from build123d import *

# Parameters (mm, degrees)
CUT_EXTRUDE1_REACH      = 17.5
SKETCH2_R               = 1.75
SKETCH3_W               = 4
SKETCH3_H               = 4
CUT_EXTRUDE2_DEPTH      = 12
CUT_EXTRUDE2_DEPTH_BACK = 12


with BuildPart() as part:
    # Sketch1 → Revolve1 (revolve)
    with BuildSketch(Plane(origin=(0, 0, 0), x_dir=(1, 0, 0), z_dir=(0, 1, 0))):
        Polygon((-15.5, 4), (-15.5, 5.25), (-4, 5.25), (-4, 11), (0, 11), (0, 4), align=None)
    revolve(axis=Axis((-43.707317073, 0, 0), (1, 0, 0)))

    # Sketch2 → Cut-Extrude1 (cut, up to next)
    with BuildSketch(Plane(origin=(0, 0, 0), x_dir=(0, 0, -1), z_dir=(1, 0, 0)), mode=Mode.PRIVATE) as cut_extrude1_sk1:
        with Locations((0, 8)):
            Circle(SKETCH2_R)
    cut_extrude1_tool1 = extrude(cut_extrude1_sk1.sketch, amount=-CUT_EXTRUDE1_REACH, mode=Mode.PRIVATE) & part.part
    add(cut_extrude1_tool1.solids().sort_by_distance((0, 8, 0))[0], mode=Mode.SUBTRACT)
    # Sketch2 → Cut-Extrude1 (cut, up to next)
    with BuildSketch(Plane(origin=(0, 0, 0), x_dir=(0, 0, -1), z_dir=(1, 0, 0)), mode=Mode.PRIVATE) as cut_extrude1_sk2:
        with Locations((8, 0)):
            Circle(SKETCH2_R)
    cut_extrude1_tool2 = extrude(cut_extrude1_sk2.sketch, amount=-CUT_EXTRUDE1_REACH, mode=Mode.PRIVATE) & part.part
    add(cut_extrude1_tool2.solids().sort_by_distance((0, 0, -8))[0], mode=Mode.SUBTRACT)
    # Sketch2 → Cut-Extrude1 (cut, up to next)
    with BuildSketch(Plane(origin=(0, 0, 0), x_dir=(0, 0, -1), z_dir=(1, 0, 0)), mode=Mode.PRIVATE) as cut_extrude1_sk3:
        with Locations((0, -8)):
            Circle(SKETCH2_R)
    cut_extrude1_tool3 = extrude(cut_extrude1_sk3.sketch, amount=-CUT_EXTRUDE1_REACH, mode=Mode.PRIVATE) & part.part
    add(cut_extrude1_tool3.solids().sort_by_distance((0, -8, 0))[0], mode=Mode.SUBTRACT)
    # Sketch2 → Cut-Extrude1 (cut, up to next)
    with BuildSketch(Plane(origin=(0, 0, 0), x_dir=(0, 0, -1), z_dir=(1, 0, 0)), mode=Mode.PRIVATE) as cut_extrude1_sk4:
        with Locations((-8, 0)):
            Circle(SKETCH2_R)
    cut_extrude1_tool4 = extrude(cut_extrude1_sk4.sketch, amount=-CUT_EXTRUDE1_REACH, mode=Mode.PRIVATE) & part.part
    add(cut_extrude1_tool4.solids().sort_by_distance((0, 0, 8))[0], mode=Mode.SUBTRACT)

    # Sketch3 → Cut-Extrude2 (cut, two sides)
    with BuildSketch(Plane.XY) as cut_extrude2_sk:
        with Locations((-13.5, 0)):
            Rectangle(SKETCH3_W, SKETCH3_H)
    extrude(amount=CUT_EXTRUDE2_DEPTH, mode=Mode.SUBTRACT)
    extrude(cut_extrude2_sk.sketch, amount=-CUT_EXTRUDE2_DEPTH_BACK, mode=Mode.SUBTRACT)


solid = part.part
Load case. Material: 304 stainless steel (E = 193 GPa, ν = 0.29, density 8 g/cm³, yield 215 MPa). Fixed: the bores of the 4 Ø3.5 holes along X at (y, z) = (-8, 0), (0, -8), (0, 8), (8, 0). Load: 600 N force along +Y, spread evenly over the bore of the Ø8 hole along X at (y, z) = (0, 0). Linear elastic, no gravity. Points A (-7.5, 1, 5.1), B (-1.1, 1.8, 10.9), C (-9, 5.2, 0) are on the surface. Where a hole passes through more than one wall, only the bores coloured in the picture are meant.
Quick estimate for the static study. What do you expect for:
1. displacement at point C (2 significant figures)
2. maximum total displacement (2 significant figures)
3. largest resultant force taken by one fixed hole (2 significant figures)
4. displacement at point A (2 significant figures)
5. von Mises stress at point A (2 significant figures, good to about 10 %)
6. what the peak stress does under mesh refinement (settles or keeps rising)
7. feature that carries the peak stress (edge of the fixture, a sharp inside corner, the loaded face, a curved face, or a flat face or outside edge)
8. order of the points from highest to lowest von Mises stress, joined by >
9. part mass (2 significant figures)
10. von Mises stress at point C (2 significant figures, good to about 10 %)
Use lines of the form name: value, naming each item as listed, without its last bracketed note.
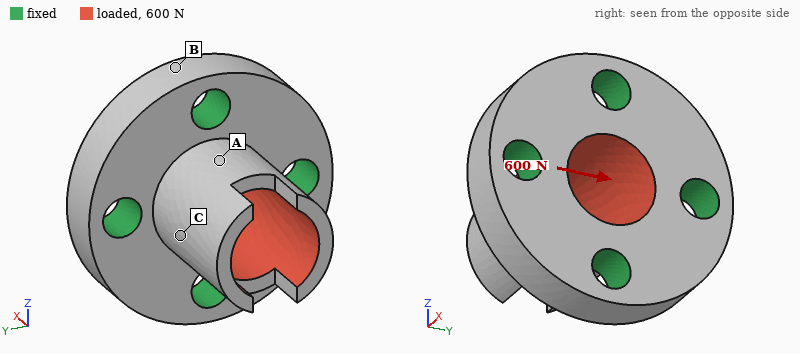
displacement at point C: 2.4 µm
maximum total displacement: 5.3 µm
largest resultant force taken by one fixed hole: 280 N
displacement at point A: 1.4 µm
von Mises stress at point A: 27 MPa
what the peak stress does under mesh refinement: keeps rising
feature that carries the peak stress: a sharp inside corner
order of the points from highest to lowest von Mises stress, joined by >: A > C > B
part mass: 12 g
von Mises stress at point C: 17 MPa
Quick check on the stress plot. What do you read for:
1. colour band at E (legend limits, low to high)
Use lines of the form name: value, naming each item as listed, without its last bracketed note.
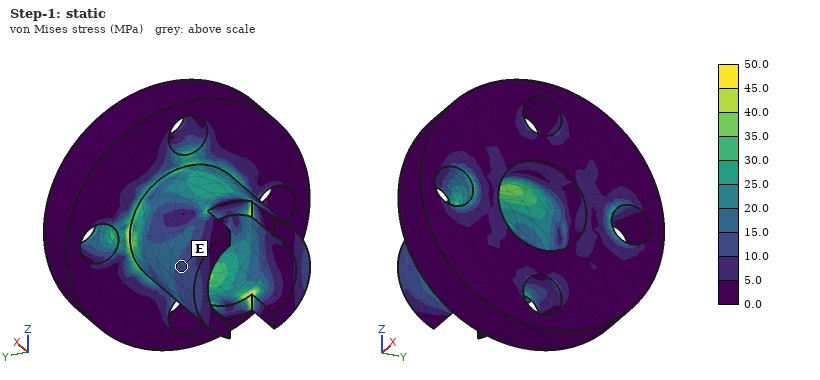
colour band at E: 10.0 to 15.0 MPa
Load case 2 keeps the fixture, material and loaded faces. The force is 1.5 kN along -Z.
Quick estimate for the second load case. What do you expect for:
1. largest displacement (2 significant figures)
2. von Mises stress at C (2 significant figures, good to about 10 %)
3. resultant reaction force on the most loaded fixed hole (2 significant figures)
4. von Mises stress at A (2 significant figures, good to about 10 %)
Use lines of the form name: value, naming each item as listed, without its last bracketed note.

largest displacement: 14 µm
von Mises stress at C: 34 MPa
resultant reaction force on the most loaded fixed hole: 690 N
von Mises stress at A: 23 MPa
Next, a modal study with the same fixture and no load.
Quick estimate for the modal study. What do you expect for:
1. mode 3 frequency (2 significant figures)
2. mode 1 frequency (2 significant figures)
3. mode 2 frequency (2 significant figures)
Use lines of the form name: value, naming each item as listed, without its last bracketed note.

mode 3 frequency: 34 kHz
mode 1 frequency: 31 kHz
mode 2 frequency: 33 kHz
